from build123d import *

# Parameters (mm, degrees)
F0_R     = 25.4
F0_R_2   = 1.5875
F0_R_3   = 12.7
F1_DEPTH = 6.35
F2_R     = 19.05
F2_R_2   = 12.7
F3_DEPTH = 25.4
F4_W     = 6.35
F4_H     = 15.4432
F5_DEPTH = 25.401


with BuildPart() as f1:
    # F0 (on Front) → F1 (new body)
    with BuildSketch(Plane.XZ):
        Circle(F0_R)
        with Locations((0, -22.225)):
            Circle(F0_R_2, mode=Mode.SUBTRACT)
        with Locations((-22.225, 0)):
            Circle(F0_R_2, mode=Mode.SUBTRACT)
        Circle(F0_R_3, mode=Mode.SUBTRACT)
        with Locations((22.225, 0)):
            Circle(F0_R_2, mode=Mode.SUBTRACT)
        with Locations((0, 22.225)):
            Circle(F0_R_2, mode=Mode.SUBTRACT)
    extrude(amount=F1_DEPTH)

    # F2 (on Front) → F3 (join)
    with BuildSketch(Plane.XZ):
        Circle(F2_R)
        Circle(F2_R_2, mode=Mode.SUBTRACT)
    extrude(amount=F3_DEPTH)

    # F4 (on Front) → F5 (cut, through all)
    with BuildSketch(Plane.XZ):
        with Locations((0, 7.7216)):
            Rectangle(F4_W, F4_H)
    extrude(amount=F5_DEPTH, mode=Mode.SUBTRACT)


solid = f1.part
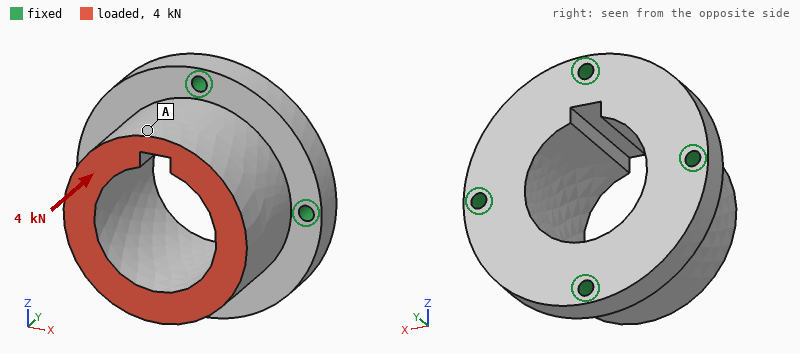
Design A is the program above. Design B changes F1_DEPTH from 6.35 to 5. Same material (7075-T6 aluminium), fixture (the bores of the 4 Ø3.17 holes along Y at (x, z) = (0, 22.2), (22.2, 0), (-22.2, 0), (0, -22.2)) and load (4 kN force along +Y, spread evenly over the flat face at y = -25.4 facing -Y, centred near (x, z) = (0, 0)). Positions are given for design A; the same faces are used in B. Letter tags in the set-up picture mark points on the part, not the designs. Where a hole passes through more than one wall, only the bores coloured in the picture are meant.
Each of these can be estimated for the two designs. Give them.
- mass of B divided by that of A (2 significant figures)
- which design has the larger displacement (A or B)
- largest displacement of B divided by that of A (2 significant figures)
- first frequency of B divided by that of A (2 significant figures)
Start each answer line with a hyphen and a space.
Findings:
- 0.95
- B
- 1.2
- 0.87
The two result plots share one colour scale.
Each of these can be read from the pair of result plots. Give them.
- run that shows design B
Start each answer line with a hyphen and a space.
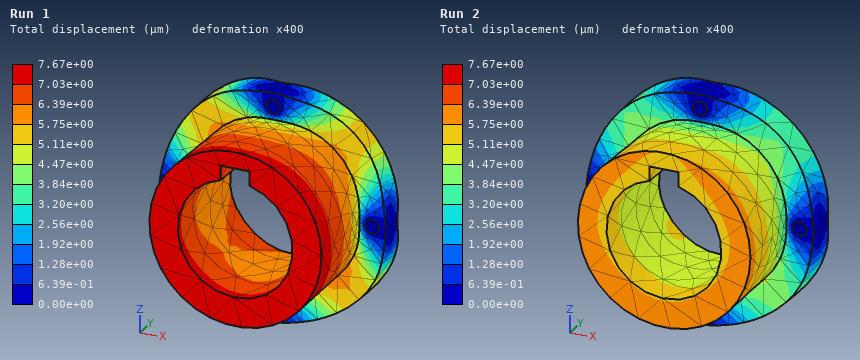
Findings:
- Run 1
